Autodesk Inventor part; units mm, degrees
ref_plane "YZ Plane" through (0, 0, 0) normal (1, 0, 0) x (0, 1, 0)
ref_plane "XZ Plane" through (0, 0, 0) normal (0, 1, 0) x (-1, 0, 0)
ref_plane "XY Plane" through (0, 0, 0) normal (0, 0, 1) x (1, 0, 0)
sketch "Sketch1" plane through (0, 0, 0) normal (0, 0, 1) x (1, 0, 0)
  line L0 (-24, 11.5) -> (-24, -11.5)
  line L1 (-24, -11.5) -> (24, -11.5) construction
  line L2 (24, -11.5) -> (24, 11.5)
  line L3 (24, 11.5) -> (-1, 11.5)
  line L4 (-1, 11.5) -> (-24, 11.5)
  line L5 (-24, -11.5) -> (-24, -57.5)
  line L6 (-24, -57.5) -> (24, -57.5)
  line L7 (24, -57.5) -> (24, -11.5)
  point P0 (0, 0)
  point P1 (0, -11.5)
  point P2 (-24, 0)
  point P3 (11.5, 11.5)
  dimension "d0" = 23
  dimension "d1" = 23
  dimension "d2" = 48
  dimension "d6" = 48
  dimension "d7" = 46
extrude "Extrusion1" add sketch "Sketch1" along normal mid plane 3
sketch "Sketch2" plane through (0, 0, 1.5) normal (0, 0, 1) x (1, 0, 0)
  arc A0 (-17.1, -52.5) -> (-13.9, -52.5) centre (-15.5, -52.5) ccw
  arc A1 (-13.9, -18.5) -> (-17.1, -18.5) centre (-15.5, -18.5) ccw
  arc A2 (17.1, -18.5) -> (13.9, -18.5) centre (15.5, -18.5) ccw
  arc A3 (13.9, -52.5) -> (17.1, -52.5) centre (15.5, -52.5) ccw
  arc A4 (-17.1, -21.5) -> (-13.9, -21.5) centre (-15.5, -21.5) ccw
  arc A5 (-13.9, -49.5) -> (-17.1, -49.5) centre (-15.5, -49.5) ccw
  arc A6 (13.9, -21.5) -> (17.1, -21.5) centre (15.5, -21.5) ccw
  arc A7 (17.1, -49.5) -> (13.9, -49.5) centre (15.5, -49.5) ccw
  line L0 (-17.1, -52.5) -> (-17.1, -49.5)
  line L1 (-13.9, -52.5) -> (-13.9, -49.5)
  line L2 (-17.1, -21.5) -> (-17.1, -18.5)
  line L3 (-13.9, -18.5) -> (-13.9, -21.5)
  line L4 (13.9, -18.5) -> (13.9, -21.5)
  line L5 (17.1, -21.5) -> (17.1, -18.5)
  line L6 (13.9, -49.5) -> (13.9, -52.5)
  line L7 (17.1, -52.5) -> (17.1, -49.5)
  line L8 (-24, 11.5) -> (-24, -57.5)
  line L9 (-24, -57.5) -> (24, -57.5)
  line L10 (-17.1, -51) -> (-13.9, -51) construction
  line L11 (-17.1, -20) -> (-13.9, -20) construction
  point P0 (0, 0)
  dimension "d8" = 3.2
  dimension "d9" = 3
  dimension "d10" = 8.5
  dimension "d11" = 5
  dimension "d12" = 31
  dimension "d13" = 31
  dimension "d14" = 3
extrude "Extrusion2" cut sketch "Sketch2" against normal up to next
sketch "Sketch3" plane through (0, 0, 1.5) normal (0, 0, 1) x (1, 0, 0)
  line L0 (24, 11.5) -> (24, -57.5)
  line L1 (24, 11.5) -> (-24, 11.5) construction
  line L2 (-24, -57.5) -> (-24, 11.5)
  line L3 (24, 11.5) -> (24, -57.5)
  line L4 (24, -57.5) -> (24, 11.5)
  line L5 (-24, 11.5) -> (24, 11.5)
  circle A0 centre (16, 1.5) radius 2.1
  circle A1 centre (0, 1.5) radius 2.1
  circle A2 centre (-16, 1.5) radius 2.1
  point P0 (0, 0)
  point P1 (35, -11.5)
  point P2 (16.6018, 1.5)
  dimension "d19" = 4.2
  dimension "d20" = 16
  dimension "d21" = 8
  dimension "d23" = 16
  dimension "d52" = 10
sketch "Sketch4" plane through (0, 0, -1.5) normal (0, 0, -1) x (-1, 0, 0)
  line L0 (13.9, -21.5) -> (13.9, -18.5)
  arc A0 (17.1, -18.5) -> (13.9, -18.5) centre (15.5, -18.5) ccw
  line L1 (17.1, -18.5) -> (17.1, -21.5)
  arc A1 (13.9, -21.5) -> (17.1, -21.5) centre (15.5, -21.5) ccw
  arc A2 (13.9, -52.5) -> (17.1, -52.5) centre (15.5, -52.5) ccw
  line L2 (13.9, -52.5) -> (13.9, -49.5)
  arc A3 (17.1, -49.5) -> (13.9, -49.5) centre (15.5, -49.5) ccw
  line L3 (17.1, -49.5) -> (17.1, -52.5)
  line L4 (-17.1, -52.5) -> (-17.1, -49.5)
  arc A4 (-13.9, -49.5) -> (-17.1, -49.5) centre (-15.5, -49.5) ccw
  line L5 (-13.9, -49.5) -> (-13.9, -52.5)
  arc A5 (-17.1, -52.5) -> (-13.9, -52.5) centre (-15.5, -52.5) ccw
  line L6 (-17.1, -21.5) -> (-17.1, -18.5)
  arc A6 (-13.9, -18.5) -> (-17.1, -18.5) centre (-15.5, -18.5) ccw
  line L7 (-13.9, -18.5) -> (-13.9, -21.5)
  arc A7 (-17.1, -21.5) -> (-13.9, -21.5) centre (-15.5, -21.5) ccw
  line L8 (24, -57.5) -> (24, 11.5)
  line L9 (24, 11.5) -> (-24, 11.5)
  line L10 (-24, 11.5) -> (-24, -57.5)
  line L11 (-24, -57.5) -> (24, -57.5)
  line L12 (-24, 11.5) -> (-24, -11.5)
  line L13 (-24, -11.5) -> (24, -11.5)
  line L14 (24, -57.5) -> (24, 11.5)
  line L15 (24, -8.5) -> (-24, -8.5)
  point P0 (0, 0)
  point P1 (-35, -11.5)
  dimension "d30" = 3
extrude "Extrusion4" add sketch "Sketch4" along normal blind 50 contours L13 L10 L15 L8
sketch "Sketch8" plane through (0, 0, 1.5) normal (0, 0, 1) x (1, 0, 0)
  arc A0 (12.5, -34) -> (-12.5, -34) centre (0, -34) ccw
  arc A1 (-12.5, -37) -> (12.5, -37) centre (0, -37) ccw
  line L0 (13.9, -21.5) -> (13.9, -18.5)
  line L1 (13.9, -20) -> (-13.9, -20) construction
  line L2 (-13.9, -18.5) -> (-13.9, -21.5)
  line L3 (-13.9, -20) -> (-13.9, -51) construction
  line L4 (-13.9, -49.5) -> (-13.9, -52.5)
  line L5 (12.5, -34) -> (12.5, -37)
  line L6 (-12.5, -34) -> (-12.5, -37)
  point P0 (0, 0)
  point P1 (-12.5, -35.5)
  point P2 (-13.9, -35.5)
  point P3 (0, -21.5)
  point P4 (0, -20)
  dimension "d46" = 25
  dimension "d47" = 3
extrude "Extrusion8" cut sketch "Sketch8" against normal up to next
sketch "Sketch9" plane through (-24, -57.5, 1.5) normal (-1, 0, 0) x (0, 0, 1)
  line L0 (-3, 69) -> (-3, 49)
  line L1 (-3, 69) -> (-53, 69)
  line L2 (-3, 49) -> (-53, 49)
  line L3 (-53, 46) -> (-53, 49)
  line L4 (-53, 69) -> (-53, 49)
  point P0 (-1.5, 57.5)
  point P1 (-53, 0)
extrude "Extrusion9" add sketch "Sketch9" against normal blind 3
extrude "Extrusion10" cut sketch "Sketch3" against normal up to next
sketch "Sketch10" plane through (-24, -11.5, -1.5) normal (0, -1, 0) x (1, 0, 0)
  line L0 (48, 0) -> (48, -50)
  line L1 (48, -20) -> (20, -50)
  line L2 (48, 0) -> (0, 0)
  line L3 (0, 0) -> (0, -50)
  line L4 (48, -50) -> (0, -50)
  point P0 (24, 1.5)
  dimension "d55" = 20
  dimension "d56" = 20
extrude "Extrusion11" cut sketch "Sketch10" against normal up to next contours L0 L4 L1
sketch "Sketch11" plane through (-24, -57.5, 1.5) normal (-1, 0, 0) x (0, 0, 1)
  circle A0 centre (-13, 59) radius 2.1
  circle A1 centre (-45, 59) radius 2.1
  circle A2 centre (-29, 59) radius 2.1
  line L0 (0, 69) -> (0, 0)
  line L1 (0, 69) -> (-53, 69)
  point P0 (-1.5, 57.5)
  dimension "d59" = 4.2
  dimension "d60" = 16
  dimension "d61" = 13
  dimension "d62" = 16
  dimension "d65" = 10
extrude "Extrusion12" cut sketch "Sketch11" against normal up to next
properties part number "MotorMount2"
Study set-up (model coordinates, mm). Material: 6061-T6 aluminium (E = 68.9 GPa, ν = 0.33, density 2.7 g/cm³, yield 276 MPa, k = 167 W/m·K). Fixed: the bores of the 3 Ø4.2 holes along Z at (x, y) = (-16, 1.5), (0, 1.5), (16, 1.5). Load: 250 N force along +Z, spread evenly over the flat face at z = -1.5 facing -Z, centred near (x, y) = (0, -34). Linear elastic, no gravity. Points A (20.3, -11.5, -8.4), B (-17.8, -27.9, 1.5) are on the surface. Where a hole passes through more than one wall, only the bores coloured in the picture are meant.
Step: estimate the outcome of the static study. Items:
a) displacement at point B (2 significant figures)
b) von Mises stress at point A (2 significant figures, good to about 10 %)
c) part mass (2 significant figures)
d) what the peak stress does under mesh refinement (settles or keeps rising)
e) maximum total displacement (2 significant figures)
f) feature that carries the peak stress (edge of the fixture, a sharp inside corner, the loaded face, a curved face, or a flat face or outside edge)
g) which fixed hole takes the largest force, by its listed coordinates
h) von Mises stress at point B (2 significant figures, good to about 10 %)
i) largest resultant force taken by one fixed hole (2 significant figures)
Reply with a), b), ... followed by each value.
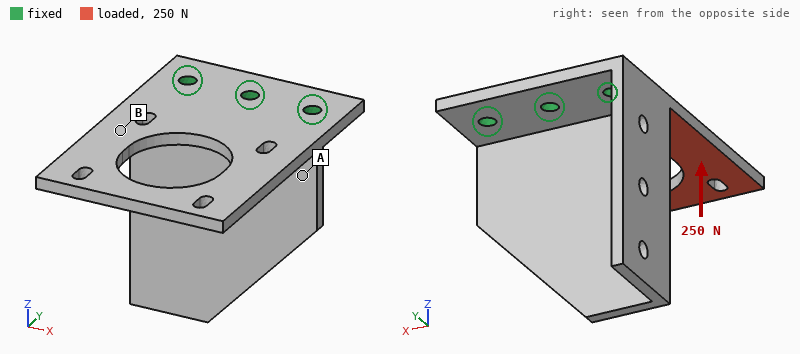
a) 0.26 mm
b) 13 MPa
c) 45 g
d) keeps rising
e) 1.0 mm
f) edge of the fixture
g) (0, 1.5)
h) 65 MPa
i) 120 N
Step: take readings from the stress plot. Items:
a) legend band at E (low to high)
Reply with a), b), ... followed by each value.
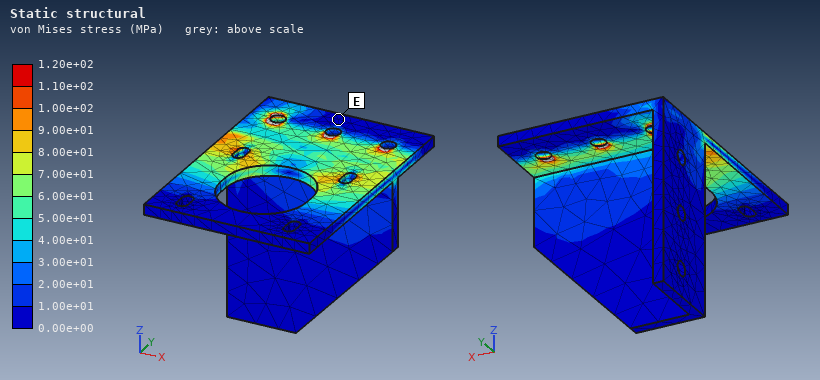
a) 0.00e+00 to 1.00e+01 MPa
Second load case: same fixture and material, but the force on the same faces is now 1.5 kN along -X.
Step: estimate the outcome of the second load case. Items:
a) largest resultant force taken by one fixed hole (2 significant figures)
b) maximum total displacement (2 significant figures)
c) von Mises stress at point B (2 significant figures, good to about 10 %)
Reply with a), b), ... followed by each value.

a) 1.6 kN
b) 0.19 mm
c) 18 MPa
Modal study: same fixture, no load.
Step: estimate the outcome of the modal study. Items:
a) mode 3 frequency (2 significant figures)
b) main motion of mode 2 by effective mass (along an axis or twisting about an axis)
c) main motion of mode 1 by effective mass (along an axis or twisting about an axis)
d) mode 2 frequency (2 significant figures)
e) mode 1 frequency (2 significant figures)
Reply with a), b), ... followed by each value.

a) 1900 Hz
b) along Y
c) along Z
d) 1500 Hz
e) 810 Hz
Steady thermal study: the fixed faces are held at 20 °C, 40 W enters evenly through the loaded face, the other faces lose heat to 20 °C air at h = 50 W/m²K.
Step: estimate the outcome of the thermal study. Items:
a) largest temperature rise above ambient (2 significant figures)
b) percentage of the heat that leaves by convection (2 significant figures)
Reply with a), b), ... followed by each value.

a) 69 K
b) 23 %
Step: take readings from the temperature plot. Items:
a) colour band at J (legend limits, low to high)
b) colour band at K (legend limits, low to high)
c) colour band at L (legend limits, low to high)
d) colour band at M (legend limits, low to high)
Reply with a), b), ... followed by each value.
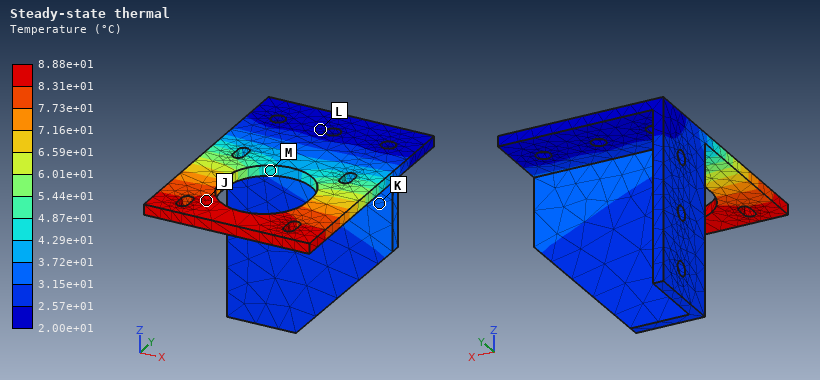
a) 8.31e+01 to 8.88e+01 °C
b) 3.15e+01 to 3.72e+01 °C
c) 2.00e+01 to 2.57e+01 °C
d) 4.29e+01 to 4.87e+01 °C
